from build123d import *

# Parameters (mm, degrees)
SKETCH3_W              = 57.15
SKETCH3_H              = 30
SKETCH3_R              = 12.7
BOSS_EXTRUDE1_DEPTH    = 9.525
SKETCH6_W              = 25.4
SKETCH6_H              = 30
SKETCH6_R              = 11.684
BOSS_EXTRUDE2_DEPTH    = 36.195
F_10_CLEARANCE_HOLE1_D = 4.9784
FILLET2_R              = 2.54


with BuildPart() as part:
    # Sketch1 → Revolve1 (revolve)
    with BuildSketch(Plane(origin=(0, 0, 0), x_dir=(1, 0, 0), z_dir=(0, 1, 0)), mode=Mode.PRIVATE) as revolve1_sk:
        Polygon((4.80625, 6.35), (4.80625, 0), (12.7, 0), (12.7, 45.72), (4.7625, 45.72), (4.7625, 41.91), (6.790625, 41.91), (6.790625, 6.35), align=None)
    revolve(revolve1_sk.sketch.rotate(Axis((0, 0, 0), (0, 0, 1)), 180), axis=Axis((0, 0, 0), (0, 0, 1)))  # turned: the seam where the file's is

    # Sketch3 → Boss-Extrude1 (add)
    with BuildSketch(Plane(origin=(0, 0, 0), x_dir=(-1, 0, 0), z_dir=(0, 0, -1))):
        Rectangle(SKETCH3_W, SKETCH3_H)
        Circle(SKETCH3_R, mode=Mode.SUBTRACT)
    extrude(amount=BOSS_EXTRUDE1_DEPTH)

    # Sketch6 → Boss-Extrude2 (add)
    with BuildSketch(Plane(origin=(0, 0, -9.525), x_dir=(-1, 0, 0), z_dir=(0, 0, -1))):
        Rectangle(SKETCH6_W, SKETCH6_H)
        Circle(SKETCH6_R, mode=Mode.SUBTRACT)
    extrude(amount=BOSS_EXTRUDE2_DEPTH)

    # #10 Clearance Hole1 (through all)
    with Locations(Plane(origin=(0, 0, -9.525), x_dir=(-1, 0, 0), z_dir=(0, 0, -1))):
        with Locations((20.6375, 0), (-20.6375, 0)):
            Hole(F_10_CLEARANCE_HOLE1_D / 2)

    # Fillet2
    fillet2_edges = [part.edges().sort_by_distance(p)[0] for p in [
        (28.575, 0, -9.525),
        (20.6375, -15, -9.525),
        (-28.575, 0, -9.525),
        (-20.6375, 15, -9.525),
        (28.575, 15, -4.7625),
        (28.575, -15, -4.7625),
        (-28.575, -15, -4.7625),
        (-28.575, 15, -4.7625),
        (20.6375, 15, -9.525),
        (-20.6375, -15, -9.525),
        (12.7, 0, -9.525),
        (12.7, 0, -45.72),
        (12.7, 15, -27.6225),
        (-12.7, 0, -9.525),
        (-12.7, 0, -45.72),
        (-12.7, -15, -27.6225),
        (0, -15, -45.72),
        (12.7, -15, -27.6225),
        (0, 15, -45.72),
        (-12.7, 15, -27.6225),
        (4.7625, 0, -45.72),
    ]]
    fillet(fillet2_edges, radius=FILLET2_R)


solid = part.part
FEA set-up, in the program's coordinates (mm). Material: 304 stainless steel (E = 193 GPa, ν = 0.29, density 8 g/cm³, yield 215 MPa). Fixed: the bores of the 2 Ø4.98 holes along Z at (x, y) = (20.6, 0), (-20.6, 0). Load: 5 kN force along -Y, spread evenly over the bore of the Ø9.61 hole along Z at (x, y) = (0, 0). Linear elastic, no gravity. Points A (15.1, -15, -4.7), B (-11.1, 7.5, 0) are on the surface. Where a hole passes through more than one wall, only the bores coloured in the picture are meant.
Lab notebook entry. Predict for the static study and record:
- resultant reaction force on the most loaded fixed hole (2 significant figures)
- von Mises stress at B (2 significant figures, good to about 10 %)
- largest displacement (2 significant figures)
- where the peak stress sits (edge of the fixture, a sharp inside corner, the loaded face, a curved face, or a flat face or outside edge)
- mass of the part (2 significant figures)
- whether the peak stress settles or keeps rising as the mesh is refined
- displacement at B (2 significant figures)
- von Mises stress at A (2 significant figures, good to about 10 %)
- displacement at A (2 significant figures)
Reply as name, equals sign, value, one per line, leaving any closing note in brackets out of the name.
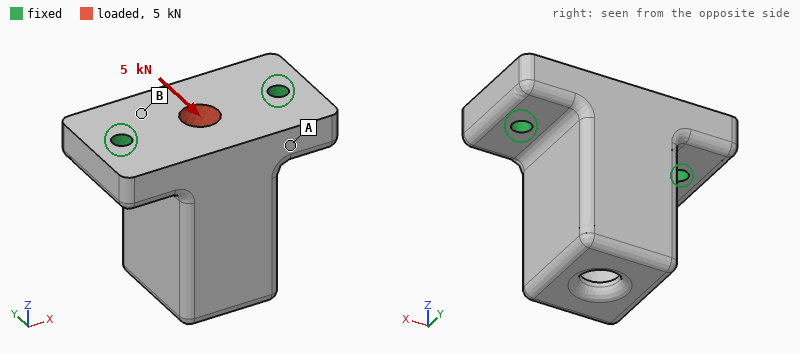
resultant reaction force on the most loaded fixed hole = 2.5 kN
von Mises stress at B = 20 MPa
largest displacement = 4.4 µm
where the peak stress sits = edge of the fixture
mass of the part = 300 g
whether the peak stress settles or keeps rising as the mesh is refined = keeps rising
displacement at B = 2.4 µm
von Mises stress at A = 5.6 MPa
displacement at A = 2.0 µm
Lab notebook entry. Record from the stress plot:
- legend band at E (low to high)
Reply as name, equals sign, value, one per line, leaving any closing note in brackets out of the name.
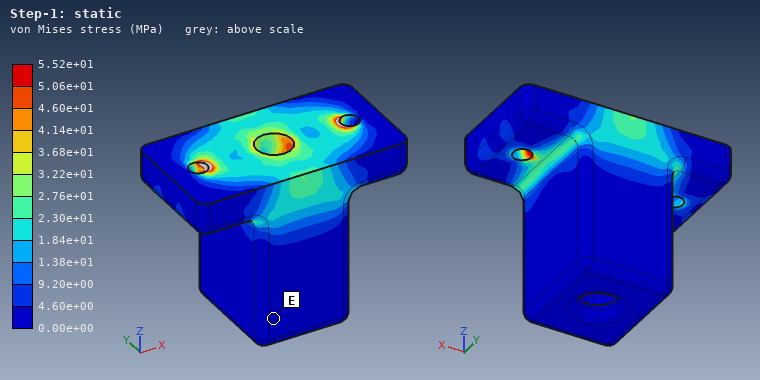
legend band at E = 0.00e+00 to 4.60e+00 MPa
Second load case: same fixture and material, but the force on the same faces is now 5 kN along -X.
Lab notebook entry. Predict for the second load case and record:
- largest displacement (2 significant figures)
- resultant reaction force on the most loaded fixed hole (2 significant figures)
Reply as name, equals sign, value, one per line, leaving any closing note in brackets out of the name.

largest displacement = 2.0 µm
resultant reaction force on the most loaded fixed hole = 2.5 kN
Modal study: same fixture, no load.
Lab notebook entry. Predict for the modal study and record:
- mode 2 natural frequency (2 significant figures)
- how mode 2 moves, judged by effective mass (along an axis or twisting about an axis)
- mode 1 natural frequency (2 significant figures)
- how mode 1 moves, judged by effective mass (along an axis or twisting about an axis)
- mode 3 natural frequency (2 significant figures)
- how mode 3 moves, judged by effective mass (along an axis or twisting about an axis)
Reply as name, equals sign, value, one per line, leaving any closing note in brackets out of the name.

mode 2 natural frequency = 7700 Hz
how mode 2 moves, judged by effective mass = along X
mode 1 natural frequency = 3900 Hz
how mode 1 moves, judged by effective mass = along Y
mode 3 natural frequency = 12 kHz
how mode 3 moves, judged by effective mass = along Z
